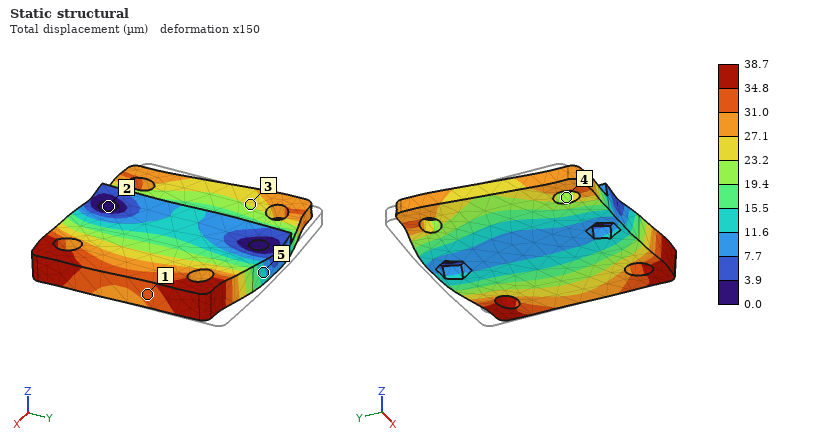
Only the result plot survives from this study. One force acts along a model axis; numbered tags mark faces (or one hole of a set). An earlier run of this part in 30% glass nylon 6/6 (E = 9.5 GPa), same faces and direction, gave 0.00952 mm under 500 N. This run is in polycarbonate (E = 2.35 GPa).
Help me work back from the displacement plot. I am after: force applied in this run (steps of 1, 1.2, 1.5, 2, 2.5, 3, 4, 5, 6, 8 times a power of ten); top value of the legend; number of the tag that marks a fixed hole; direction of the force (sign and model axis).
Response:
500 N
38.7 µm
2
-Y
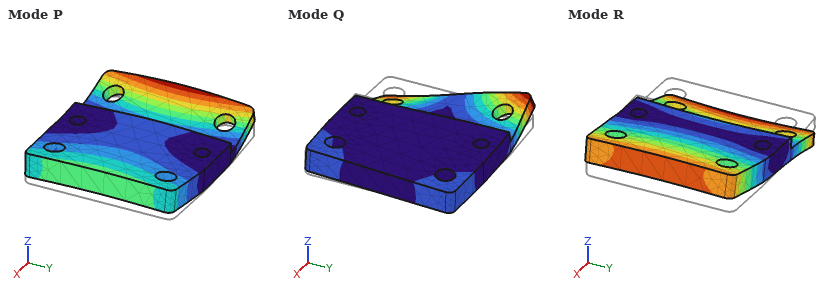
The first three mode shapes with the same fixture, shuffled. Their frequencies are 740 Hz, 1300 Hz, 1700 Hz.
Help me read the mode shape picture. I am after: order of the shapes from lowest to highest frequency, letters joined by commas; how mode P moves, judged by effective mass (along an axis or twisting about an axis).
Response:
R, P, Q
along Z
